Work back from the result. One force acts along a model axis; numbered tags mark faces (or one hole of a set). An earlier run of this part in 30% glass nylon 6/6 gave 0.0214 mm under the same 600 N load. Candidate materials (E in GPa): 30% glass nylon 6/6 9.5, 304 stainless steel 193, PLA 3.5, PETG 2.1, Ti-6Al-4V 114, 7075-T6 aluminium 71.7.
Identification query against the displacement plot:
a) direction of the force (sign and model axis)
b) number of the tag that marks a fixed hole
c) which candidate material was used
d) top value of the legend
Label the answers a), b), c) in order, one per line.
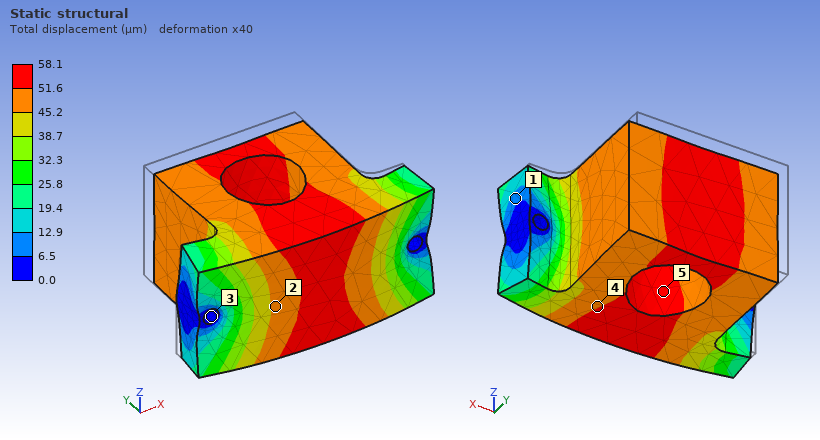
a) -Y
b) 3
c) PLA
d) 58.1 µm
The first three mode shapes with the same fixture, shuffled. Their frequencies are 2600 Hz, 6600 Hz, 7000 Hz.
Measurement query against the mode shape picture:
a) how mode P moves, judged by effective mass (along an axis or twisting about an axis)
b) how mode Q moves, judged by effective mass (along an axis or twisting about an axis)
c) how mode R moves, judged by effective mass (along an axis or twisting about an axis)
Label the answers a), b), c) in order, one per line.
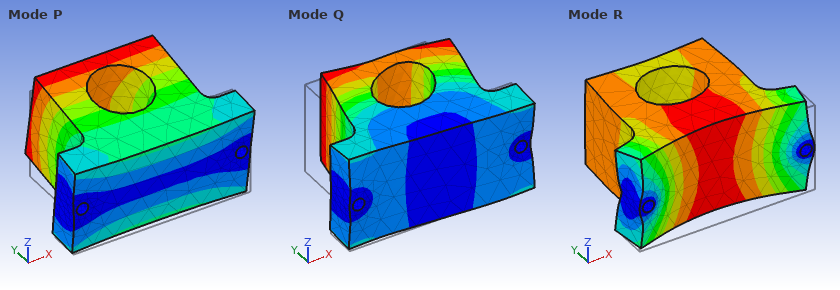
a) along Z
b) along X
c) along Y
